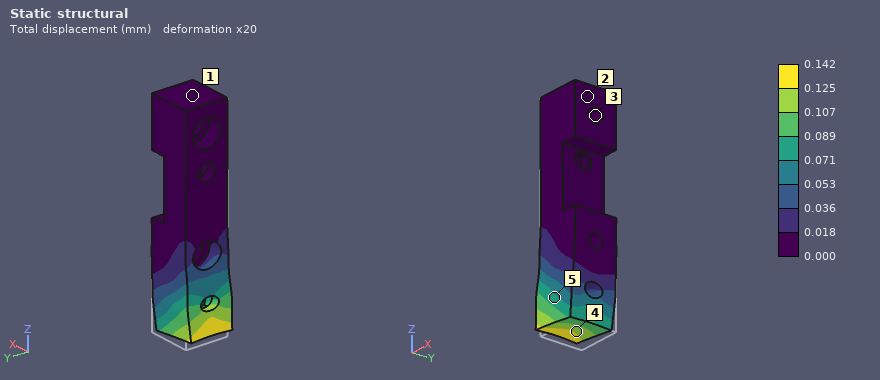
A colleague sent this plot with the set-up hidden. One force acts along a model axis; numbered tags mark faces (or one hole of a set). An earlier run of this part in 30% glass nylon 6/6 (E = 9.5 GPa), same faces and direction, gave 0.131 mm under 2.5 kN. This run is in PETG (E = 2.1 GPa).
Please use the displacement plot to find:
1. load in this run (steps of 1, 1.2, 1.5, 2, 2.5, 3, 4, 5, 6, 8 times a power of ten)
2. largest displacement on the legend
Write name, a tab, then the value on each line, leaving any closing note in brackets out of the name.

load in this run	600 N
largest displacement on the legend	0.142 mm
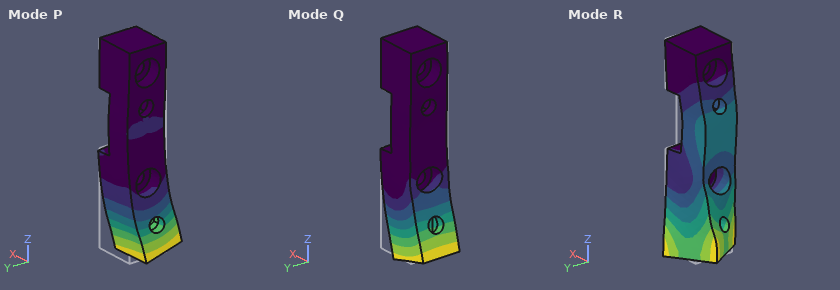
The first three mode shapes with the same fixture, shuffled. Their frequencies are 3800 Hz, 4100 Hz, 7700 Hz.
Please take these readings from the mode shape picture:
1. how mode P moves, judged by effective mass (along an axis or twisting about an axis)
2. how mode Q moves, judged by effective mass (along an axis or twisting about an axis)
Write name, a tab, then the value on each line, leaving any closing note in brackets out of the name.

how mode P moves, judged by effective mass	along Y
how mode Q moves, judged by effective mass	along X
